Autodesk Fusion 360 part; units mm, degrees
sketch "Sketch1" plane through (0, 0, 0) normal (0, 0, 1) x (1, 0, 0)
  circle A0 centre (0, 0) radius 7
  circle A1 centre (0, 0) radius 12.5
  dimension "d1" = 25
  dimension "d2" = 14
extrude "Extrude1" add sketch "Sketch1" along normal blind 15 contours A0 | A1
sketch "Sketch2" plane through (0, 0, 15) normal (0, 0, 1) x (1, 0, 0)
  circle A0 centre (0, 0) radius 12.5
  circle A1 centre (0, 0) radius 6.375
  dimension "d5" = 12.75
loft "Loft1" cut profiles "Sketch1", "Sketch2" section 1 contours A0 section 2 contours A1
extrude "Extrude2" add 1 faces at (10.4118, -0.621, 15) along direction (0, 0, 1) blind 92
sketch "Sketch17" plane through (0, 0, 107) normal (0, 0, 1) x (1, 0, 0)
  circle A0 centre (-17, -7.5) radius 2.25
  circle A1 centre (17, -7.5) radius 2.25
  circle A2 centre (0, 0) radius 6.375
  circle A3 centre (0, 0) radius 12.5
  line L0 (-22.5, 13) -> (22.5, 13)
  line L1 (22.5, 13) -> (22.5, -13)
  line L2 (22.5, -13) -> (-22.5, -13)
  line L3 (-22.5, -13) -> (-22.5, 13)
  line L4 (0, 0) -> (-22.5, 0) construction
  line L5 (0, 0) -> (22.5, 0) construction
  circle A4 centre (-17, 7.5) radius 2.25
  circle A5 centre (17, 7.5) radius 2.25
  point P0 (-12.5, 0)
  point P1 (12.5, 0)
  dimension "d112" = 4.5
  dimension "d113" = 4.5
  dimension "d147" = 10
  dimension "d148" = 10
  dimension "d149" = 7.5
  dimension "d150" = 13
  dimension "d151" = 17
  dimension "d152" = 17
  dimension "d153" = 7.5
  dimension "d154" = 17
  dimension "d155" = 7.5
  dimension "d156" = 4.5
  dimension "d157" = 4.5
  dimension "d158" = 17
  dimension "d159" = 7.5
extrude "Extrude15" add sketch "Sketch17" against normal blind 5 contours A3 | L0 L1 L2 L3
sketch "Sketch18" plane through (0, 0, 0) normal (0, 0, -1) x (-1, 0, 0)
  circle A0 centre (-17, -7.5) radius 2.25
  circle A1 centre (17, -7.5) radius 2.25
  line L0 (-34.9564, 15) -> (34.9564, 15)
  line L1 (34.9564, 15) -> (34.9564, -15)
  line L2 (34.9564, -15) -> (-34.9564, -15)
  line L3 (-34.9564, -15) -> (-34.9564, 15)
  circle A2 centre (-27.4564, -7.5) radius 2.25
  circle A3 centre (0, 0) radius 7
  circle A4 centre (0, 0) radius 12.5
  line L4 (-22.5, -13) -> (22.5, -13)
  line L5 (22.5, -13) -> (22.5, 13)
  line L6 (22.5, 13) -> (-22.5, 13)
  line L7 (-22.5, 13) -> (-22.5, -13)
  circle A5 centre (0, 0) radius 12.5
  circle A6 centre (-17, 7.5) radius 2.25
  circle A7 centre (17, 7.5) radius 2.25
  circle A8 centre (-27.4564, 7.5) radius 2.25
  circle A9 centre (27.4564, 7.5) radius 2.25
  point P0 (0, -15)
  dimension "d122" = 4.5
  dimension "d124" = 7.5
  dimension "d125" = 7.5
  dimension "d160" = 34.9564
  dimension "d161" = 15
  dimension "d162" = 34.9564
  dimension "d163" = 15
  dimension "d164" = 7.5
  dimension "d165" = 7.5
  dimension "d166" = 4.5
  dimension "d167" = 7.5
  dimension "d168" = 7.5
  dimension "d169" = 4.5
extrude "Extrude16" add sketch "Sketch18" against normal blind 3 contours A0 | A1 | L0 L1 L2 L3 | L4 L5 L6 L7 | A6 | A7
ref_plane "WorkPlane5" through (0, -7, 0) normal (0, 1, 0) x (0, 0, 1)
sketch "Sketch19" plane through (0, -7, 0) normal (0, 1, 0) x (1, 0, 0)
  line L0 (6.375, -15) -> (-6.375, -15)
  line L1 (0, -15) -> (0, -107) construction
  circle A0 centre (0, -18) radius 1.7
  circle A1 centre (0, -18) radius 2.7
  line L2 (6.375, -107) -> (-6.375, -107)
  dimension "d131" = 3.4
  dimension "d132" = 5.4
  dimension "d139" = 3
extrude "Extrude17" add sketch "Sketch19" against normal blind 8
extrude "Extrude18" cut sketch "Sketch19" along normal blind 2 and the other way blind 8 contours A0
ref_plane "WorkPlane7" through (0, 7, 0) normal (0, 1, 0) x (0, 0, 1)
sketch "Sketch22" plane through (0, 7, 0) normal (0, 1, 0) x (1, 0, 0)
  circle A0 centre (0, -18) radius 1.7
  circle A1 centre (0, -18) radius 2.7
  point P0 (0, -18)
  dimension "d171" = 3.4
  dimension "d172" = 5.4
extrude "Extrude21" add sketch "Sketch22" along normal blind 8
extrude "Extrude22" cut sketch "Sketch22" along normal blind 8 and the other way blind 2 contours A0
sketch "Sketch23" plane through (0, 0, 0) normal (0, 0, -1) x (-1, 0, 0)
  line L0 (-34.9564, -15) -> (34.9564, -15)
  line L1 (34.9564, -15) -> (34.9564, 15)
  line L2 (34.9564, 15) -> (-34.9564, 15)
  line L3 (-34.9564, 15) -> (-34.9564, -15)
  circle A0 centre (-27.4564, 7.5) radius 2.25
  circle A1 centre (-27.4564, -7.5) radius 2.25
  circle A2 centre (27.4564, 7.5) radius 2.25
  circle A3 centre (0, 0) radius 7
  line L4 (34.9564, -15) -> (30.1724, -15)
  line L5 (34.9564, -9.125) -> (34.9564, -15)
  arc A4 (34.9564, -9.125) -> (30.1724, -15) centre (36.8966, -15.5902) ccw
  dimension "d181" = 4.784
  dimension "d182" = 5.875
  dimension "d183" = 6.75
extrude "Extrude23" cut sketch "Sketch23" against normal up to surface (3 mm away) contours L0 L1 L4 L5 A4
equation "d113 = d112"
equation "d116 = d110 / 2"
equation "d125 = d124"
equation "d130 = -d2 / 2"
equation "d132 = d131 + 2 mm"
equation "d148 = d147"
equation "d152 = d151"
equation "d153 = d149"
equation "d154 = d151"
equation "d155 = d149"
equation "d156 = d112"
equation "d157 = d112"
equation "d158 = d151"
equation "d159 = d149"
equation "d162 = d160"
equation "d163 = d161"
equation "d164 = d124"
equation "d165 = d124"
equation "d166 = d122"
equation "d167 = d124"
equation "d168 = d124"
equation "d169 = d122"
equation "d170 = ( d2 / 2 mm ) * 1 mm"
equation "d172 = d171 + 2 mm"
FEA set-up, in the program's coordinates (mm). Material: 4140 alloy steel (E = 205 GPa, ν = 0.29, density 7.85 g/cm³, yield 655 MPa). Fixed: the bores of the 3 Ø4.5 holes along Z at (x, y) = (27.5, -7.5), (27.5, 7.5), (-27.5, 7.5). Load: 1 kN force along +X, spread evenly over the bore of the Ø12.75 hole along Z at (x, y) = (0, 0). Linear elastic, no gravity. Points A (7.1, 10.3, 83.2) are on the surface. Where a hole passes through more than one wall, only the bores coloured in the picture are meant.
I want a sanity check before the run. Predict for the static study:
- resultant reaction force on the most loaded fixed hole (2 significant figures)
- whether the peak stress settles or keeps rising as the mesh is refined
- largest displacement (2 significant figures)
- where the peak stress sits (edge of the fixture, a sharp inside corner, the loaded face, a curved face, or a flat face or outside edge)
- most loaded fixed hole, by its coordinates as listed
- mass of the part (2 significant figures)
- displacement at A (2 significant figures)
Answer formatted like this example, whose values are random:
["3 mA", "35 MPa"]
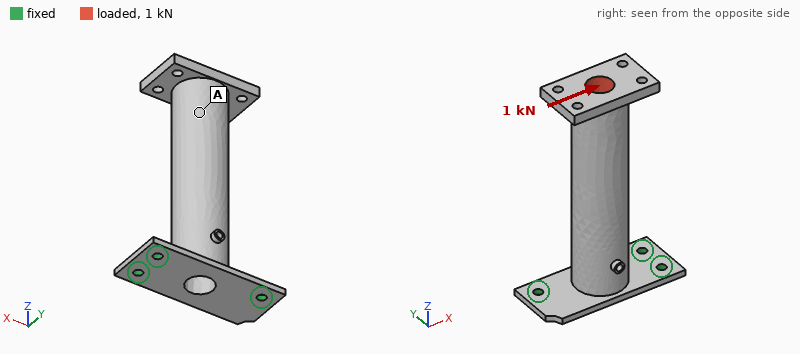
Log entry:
["1.5 kN", "keeps rising", "0.47 mm", "edge of the fixture", "(-27.5, 7.5)", "360 g", "0.35 mm"]
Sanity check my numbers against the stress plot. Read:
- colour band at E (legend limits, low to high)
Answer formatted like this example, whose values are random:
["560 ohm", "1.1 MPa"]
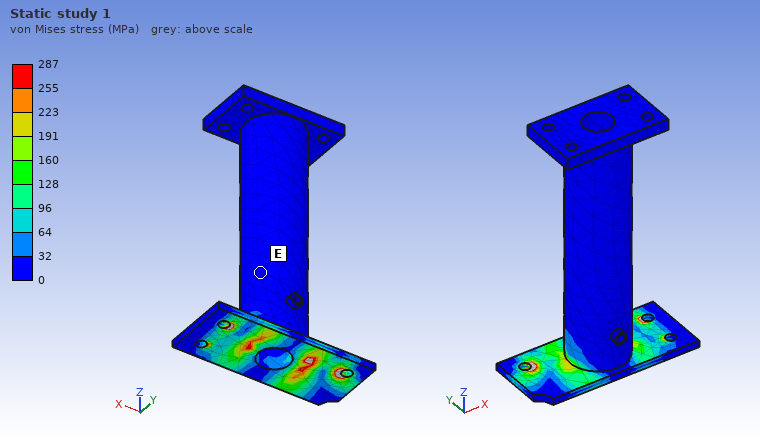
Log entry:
["0 to 32 MPa"]
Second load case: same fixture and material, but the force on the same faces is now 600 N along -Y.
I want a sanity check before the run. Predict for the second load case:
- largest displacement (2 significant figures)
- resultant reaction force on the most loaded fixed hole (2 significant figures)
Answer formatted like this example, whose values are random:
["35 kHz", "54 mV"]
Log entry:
["1.1 mm", "1.5 kN"]
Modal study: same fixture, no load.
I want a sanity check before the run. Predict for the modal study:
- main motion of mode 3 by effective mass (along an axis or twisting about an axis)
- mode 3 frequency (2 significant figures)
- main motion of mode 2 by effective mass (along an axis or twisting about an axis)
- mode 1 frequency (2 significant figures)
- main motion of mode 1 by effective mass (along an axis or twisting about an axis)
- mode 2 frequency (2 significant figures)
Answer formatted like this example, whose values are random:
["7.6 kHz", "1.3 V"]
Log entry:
["along Z", "1900 Hz", "along X", "260 Hz", "along Y", "540 Hz"]
